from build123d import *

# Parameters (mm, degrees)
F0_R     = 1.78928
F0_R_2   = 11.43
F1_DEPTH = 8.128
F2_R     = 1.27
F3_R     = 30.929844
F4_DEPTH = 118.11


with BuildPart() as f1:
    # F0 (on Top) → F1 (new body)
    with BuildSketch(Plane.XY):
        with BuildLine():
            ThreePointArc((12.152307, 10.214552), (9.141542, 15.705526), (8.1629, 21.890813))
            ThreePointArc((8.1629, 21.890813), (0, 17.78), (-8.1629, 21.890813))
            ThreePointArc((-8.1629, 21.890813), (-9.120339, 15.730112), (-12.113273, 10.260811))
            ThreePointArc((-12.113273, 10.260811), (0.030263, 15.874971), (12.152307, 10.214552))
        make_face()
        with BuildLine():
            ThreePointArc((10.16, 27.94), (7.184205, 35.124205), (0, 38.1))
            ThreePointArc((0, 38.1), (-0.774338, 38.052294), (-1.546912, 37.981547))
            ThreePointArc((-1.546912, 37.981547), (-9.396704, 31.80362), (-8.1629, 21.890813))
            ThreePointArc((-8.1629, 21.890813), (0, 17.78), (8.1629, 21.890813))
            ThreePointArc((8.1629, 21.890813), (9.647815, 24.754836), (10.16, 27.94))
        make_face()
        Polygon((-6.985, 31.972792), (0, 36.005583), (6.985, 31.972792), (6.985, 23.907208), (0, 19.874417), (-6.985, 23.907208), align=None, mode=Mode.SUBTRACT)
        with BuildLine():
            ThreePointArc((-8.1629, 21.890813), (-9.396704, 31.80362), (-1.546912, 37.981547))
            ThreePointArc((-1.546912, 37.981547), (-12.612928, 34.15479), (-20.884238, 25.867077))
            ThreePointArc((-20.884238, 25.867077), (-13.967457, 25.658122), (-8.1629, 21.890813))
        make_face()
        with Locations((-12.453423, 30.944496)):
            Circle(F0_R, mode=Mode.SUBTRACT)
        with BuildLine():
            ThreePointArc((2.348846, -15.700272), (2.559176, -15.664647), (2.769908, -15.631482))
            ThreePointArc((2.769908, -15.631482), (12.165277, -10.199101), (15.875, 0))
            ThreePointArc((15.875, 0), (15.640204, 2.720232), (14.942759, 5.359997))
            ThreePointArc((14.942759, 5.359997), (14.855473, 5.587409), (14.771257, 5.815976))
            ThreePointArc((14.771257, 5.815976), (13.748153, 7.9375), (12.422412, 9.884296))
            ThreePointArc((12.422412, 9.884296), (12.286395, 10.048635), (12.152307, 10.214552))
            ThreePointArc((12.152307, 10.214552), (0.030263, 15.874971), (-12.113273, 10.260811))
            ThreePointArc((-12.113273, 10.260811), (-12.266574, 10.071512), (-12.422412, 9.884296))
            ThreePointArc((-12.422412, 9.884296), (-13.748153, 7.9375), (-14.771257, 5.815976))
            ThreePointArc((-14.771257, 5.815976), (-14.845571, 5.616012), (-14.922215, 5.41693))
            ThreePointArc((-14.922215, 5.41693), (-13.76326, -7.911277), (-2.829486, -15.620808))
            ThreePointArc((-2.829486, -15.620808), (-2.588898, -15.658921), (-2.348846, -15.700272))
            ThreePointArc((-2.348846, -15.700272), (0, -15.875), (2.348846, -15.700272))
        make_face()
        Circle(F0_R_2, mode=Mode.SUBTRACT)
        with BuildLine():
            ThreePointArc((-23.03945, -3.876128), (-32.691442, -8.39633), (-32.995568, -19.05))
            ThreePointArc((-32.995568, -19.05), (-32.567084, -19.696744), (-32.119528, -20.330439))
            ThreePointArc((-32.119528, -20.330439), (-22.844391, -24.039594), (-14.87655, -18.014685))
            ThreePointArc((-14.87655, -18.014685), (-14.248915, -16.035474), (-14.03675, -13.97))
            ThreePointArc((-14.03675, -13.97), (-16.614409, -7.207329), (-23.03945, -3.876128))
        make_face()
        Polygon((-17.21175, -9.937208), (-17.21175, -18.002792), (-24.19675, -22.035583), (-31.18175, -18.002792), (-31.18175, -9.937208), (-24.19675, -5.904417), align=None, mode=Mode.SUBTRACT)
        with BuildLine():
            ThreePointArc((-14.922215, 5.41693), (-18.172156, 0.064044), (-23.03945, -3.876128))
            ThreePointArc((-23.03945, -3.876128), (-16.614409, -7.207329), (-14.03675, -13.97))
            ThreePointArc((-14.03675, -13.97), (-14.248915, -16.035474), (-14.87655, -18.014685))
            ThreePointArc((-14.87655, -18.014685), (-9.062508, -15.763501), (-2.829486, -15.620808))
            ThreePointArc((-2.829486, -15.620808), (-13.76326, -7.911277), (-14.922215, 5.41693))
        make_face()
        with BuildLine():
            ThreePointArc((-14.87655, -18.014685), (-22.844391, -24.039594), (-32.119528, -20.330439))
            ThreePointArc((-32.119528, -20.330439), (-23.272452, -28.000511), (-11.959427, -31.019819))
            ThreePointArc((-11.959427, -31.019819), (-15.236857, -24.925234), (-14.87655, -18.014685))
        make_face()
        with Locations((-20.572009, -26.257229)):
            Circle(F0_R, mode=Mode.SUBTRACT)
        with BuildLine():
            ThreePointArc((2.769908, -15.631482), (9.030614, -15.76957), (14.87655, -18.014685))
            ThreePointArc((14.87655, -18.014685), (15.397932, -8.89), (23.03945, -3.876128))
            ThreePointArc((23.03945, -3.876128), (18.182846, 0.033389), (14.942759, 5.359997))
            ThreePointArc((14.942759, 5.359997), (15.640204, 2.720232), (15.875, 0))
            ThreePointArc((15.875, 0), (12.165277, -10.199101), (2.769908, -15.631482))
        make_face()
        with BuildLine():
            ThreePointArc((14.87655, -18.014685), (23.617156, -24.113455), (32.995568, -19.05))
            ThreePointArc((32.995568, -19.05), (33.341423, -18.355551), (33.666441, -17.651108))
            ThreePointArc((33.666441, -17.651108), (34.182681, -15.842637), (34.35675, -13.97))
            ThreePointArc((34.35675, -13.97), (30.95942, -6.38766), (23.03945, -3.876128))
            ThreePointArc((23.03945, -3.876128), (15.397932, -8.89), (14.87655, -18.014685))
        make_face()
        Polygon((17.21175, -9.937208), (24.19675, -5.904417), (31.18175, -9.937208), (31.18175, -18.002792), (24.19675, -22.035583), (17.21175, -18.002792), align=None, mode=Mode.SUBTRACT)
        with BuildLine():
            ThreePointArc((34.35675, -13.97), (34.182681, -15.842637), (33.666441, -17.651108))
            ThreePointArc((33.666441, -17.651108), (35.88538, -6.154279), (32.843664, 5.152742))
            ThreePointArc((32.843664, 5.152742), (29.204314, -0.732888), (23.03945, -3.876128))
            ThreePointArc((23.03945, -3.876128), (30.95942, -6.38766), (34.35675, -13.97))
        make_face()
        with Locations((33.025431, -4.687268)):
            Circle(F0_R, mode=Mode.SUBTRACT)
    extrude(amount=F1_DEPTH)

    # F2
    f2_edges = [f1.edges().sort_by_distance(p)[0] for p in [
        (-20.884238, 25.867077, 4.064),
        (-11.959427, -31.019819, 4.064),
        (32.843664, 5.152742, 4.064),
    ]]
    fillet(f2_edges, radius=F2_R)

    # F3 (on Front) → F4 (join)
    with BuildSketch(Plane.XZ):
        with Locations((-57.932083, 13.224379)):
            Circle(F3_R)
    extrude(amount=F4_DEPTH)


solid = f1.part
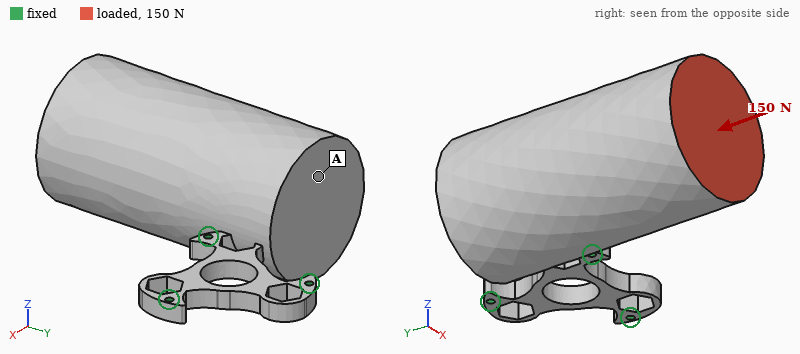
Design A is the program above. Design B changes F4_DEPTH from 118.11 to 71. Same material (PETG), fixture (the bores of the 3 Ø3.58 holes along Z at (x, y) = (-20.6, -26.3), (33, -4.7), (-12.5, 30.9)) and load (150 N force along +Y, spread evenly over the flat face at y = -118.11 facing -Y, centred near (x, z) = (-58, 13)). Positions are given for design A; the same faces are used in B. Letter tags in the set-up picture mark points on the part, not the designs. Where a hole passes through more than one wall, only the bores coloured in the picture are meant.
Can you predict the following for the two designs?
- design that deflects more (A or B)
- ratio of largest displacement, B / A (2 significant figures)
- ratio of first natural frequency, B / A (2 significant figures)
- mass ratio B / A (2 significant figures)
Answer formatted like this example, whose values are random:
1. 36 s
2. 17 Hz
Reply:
1. A
2. 0.69
3. 1.6
4. 0.61
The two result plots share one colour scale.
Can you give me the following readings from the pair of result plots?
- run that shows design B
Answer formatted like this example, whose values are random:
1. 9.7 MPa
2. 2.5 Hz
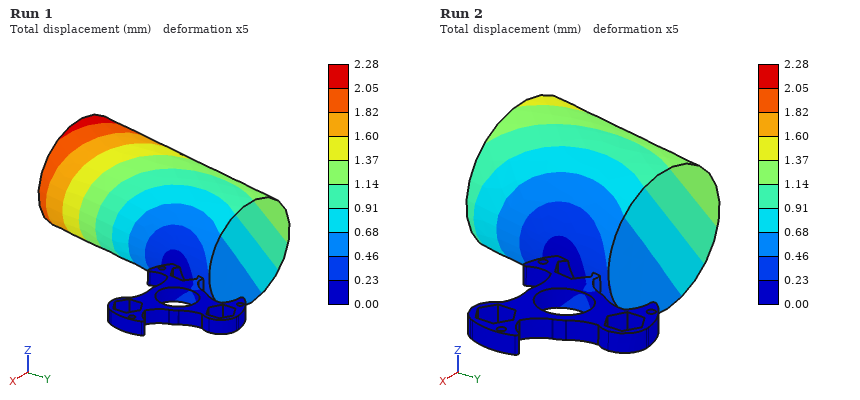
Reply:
1. Run 2
